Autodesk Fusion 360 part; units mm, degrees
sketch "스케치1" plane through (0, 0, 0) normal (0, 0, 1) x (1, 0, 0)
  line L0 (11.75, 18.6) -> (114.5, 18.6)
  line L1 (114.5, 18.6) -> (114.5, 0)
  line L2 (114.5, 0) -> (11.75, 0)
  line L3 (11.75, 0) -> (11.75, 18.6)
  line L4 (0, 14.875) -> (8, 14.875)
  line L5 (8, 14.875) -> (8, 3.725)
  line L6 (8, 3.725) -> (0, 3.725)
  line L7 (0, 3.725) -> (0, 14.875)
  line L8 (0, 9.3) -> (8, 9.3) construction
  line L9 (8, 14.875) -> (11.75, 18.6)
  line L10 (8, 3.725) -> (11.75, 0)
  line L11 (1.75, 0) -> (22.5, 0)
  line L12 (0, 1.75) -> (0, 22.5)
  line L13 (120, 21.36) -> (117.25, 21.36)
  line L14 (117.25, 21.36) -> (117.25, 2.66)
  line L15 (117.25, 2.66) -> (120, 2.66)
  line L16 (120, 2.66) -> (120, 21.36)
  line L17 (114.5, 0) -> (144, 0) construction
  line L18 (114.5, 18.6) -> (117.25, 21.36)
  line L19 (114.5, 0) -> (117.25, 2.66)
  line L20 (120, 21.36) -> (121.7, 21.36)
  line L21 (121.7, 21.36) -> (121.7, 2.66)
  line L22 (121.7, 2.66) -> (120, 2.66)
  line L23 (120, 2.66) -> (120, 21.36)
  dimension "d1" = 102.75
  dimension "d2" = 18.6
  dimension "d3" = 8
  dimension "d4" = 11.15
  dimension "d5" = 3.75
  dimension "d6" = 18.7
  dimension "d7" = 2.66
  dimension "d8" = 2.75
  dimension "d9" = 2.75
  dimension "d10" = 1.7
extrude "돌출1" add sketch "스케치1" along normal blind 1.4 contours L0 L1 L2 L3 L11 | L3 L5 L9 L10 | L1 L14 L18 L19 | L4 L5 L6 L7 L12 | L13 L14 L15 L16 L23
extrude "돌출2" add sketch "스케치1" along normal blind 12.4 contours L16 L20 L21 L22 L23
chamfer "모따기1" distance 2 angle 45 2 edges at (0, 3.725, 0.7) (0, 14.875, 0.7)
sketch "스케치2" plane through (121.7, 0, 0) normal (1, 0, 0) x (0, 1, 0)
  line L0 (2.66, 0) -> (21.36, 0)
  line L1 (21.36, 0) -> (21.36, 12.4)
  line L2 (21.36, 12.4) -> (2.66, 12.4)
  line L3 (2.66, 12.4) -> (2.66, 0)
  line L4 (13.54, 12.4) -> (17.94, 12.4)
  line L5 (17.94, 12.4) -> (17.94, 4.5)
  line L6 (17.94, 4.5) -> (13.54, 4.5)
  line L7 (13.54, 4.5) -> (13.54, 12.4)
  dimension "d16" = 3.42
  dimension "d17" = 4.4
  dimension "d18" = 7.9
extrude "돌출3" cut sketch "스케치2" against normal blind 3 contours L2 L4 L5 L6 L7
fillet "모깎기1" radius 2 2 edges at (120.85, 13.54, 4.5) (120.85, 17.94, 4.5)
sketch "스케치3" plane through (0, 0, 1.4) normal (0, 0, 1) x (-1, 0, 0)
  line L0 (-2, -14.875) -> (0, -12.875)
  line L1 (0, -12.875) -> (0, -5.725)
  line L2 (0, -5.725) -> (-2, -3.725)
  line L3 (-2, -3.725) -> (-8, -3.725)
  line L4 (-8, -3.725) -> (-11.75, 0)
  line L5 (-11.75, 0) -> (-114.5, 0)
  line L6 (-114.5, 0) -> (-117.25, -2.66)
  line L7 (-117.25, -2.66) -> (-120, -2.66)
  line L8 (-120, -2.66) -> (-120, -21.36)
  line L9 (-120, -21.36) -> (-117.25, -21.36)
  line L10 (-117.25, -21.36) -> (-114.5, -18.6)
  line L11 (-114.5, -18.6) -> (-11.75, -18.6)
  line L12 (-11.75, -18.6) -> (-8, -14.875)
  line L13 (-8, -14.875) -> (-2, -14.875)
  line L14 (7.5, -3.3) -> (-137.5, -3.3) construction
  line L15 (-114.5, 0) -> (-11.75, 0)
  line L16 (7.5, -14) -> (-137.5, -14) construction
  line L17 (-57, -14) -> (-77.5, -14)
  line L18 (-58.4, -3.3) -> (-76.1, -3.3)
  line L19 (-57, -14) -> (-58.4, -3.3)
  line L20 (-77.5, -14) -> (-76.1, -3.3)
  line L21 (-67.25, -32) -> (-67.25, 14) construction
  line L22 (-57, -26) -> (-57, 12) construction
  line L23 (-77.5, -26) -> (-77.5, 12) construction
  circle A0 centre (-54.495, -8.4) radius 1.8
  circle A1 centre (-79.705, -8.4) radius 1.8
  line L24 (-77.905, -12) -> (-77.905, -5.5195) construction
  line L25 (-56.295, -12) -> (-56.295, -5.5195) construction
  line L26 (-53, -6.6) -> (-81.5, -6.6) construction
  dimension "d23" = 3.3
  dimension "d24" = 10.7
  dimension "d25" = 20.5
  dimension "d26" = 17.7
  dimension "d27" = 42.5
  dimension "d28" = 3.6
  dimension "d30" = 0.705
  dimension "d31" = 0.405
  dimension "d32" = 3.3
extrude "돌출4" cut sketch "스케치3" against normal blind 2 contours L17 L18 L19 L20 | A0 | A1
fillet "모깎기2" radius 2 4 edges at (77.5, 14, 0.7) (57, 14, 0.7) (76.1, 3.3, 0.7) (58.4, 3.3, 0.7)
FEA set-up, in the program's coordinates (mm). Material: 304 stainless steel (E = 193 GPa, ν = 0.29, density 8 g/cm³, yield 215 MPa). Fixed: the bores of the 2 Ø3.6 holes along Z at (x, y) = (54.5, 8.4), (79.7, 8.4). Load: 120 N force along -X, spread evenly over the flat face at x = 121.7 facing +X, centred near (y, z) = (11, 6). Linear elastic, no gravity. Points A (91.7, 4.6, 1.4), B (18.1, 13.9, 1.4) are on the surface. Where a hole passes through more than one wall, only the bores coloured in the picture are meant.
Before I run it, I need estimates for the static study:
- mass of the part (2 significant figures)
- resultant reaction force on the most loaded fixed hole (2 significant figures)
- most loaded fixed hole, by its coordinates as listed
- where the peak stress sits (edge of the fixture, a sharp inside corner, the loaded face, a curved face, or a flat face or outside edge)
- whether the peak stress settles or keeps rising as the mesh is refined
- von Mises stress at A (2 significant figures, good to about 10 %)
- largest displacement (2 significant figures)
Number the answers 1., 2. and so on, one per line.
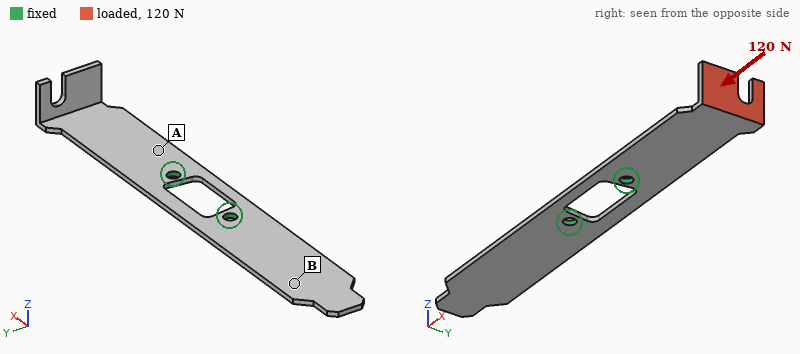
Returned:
1. 24 g
2. 100 N
3. (79.7, 8.4)
4. edge of the fixture
5. keeps rising
6. 100 MPa
7. 0.74 mm
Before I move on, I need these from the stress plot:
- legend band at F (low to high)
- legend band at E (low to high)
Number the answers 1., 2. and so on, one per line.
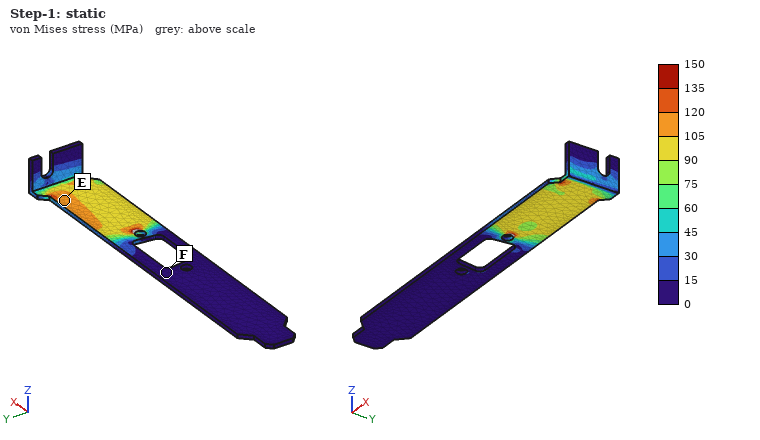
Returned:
1. 0 to 15 MPa
2. 105 to 120 MPa
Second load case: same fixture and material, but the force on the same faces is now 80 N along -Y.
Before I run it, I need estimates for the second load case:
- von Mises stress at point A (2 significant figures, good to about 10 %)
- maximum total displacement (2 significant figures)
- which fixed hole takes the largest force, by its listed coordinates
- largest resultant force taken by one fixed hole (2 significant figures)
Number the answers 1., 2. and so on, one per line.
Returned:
1. 67 MPa
2. 0.24 mm
3. (79.7, 8.4)
4. 110 N
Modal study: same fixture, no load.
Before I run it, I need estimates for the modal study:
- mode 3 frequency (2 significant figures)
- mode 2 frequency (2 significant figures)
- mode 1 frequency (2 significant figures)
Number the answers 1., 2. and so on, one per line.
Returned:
1. 1700 Hz
2. 450 Hz
3. 440 Hz
